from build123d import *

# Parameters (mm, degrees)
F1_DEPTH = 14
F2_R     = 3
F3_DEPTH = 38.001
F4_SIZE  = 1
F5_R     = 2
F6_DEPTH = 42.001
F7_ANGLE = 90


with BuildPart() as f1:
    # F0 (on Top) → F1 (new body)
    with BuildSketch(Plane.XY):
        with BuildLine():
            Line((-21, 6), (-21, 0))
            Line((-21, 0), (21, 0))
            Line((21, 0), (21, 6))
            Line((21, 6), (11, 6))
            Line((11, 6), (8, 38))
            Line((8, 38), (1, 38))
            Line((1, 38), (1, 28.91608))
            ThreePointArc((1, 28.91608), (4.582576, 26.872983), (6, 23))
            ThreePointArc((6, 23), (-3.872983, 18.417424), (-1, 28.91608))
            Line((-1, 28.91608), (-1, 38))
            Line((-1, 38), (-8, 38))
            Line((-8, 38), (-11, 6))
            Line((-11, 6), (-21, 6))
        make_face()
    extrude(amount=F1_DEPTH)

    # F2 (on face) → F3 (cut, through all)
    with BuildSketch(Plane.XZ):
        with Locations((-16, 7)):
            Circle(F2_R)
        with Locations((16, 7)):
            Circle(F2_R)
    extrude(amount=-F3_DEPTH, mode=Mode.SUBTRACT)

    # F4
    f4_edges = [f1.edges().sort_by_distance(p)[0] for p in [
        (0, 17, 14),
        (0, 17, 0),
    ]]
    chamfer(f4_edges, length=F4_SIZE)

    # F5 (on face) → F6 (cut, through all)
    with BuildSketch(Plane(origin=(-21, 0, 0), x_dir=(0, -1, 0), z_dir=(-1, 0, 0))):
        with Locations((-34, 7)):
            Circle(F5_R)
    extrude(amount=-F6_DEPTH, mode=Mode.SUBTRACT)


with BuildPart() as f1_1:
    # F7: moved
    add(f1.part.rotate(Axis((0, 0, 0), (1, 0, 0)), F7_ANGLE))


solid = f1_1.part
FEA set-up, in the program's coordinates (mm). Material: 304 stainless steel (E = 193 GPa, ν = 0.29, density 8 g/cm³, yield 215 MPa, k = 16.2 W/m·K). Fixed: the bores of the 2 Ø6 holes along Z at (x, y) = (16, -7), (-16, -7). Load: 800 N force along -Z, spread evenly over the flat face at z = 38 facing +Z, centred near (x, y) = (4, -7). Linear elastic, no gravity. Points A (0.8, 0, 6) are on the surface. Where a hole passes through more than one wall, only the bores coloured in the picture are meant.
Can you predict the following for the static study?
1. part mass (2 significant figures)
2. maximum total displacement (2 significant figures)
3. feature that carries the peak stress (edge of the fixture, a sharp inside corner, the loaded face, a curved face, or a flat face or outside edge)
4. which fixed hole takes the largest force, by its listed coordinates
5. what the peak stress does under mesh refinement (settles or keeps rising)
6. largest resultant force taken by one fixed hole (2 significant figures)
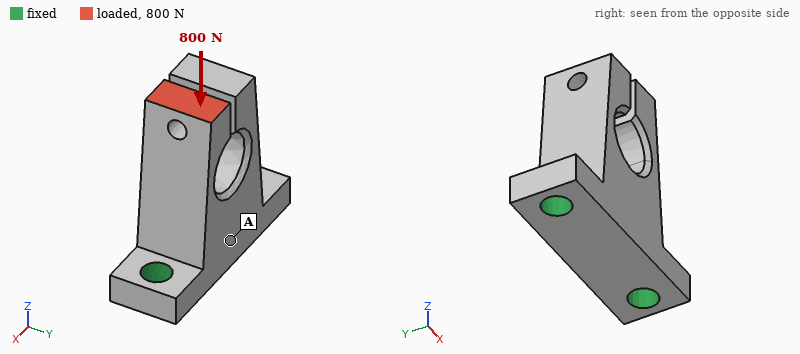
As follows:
77 g
35 µm
a sharp inside corner
(16, -7)
keeps rising
570 N
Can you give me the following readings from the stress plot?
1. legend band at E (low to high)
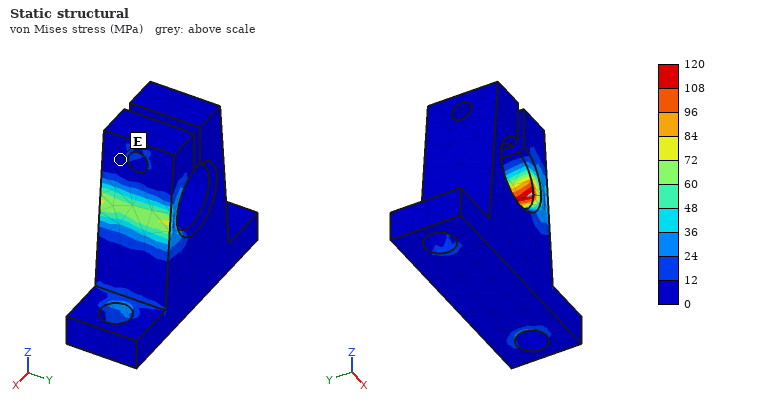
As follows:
0 to 12 MPa
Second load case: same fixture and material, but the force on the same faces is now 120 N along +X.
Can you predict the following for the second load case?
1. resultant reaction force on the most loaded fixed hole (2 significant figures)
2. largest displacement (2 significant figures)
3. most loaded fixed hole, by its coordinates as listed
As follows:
190 N
29 µm
(-16, -7)
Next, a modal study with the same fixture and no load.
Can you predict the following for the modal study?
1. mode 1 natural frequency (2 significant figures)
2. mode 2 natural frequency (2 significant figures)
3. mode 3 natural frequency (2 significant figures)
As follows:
4900 Hz
5100 Hz
5300 Hz
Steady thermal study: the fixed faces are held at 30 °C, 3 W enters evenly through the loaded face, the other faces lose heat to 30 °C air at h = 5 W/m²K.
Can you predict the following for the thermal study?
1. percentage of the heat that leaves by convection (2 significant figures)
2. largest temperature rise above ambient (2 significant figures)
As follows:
12 %
78 K
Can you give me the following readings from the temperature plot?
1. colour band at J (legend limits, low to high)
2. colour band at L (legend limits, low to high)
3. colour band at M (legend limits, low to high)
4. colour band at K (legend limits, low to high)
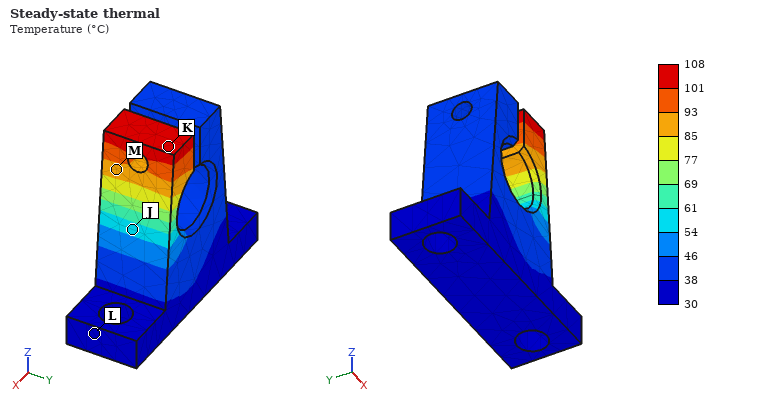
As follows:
54 to 61 °C
30 to 38 °C
85 to 93 °C
101 to 108 °C
